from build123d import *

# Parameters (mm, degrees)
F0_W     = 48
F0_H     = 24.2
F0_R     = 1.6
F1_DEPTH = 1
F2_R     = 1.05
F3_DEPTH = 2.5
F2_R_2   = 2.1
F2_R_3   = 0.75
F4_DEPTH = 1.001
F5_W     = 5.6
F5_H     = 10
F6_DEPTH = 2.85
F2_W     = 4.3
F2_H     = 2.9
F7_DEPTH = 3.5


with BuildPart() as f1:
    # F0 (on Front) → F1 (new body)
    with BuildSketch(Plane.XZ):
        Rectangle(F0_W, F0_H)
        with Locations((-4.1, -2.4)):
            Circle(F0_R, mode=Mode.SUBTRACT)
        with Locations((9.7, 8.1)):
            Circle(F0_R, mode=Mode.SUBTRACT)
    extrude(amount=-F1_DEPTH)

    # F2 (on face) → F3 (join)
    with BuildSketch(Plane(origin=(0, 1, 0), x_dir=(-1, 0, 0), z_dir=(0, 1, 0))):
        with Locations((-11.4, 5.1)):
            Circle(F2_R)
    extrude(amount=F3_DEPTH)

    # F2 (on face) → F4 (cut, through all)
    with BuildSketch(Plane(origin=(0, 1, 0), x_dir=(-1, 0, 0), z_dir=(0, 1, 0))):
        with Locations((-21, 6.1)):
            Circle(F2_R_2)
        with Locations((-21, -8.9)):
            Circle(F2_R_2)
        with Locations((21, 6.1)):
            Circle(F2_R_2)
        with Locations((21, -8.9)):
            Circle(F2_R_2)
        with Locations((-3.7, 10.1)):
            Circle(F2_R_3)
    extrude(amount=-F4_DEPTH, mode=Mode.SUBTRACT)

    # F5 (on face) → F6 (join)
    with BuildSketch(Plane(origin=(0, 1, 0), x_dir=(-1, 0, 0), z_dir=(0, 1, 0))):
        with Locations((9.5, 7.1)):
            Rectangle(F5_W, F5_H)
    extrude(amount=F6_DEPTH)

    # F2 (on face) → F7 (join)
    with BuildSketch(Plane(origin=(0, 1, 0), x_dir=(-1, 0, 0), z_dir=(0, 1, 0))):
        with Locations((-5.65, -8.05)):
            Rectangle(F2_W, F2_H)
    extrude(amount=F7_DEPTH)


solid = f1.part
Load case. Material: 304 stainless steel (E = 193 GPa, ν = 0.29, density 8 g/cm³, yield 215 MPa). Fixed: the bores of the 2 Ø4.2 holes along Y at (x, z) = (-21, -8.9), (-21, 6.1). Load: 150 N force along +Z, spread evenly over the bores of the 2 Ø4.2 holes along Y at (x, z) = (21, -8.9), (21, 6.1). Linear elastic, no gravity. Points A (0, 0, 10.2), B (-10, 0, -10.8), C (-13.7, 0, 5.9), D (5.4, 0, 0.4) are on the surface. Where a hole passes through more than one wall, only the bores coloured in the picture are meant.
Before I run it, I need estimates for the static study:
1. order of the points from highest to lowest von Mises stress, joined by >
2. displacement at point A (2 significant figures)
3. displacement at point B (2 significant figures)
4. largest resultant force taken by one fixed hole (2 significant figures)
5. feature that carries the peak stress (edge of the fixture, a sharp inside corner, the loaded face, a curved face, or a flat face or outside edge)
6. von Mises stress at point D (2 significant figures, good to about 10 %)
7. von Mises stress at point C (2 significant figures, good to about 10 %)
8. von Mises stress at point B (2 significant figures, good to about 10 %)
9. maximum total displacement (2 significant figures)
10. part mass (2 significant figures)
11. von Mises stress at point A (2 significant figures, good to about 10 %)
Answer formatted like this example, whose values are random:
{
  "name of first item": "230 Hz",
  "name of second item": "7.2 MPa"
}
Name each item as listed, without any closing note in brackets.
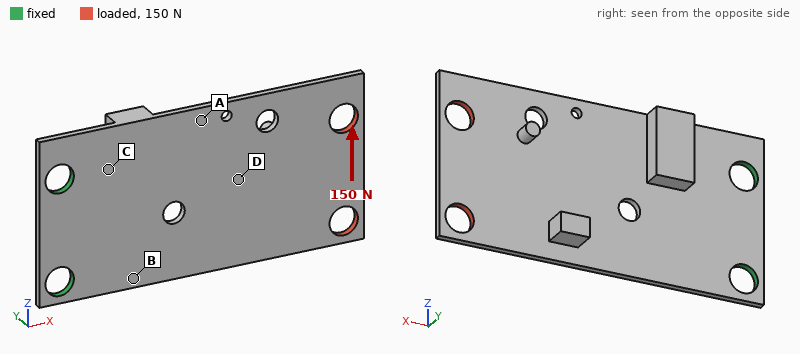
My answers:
{
  "order of the points from highest to lowest von Mises stress, joined by >": "B > C > A > D",
  "displacement at point A": "8.7 µm",
  "displacement at point B": "3.9 µm",
  "largest resultant force taken by one fixed hole": "380 N",
  "feature that carries the peak stress": "edge of the fixture",
  "von Mises stress at point D": "16 MPa",
  "von Mises stress at point C": "33 MPa",
  "von Mises stress at point B": "44 MPa",
  "maximum total displacement": "25 µm",
  "part mass": "10 g",
  "von Mises stress at point A": "24 MPa"
}
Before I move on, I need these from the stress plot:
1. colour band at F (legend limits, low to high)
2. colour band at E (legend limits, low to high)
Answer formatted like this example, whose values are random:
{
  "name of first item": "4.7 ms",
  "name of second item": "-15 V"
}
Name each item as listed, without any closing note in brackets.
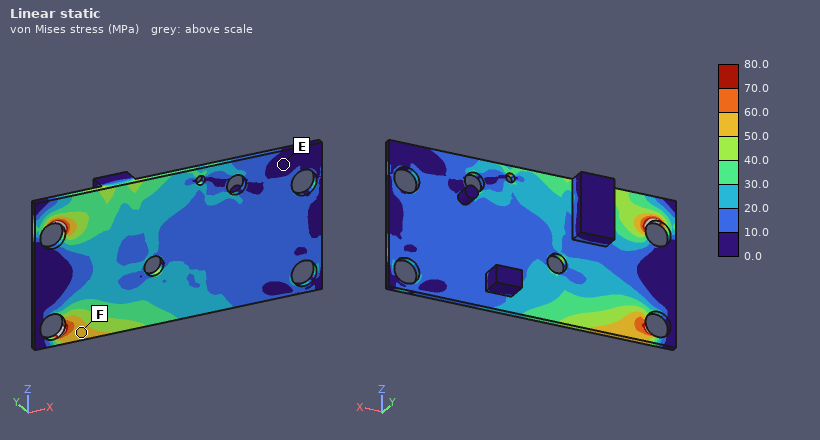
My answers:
{
  "colour band at F": "50.0 to 60.0 MPa",
  "colour band at E": "0.0 to 10.0 MPa"
}
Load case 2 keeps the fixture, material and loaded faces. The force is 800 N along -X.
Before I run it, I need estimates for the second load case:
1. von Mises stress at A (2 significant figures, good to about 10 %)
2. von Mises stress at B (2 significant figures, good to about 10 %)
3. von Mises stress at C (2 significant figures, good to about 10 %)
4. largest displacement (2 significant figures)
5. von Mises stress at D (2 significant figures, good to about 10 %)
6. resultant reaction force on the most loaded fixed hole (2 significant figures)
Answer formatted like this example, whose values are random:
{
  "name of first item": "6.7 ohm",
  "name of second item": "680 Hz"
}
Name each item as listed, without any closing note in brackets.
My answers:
{
  "von Mises stress at A": "22 MPa",
  "von Mises stress at B": "49 MPa",
  "von Mises stress at C": "35 MPa",
  "largest displacement": "19 µm",
  "von Mises stress at D": "32 MPa",
  "resultant reaction force on the most loaded fixed hole": "410 N"
}
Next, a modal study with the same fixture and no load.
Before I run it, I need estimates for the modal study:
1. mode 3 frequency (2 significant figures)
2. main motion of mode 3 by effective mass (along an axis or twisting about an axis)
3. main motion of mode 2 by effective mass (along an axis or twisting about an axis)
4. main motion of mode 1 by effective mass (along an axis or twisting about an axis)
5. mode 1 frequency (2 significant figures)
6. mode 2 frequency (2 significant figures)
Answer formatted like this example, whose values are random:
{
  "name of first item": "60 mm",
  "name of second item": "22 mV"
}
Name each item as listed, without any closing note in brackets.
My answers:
{
  "mode 3 frequency": "2500 Hz",
  "main motion of mode 3 by effective mass": "along Y",
  "main motion of mode 2 by effective mass": "twisting about X",
  "main motion of mode 1 by effective mass": "along Y",
  "mode 1 frequency": "460 Hz",
  "mode 2 frequency": "1800 Hz"
}
